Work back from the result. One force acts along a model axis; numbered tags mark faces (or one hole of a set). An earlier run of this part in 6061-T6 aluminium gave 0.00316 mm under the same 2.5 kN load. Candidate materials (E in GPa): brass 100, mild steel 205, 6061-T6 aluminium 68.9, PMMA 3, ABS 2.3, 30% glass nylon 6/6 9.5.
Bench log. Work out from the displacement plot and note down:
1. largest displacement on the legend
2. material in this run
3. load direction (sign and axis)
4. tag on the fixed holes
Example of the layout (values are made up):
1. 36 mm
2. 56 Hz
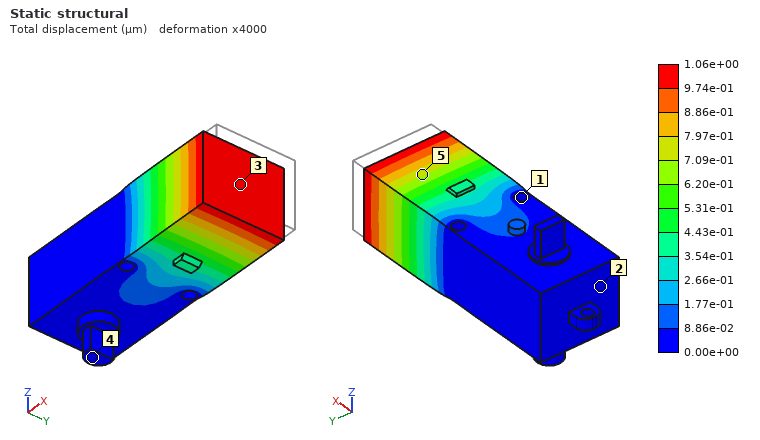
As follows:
1. 1.06e+00 µm
2. mild steel
3. -X
4. 1
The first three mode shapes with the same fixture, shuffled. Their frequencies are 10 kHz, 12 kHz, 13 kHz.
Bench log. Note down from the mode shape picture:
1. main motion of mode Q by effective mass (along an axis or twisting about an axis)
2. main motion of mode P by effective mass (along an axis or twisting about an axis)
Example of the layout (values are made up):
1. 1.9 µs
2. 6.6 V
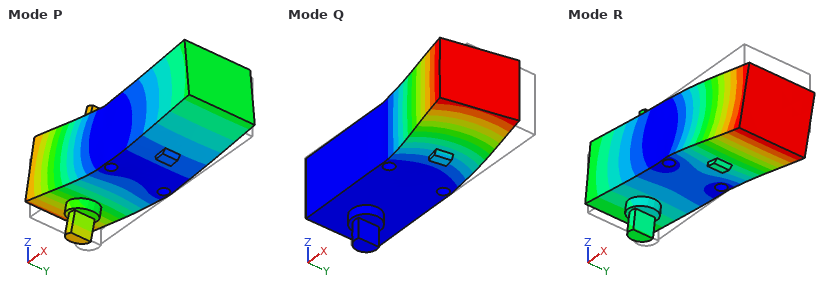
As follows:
1. along Y
2. along Z
